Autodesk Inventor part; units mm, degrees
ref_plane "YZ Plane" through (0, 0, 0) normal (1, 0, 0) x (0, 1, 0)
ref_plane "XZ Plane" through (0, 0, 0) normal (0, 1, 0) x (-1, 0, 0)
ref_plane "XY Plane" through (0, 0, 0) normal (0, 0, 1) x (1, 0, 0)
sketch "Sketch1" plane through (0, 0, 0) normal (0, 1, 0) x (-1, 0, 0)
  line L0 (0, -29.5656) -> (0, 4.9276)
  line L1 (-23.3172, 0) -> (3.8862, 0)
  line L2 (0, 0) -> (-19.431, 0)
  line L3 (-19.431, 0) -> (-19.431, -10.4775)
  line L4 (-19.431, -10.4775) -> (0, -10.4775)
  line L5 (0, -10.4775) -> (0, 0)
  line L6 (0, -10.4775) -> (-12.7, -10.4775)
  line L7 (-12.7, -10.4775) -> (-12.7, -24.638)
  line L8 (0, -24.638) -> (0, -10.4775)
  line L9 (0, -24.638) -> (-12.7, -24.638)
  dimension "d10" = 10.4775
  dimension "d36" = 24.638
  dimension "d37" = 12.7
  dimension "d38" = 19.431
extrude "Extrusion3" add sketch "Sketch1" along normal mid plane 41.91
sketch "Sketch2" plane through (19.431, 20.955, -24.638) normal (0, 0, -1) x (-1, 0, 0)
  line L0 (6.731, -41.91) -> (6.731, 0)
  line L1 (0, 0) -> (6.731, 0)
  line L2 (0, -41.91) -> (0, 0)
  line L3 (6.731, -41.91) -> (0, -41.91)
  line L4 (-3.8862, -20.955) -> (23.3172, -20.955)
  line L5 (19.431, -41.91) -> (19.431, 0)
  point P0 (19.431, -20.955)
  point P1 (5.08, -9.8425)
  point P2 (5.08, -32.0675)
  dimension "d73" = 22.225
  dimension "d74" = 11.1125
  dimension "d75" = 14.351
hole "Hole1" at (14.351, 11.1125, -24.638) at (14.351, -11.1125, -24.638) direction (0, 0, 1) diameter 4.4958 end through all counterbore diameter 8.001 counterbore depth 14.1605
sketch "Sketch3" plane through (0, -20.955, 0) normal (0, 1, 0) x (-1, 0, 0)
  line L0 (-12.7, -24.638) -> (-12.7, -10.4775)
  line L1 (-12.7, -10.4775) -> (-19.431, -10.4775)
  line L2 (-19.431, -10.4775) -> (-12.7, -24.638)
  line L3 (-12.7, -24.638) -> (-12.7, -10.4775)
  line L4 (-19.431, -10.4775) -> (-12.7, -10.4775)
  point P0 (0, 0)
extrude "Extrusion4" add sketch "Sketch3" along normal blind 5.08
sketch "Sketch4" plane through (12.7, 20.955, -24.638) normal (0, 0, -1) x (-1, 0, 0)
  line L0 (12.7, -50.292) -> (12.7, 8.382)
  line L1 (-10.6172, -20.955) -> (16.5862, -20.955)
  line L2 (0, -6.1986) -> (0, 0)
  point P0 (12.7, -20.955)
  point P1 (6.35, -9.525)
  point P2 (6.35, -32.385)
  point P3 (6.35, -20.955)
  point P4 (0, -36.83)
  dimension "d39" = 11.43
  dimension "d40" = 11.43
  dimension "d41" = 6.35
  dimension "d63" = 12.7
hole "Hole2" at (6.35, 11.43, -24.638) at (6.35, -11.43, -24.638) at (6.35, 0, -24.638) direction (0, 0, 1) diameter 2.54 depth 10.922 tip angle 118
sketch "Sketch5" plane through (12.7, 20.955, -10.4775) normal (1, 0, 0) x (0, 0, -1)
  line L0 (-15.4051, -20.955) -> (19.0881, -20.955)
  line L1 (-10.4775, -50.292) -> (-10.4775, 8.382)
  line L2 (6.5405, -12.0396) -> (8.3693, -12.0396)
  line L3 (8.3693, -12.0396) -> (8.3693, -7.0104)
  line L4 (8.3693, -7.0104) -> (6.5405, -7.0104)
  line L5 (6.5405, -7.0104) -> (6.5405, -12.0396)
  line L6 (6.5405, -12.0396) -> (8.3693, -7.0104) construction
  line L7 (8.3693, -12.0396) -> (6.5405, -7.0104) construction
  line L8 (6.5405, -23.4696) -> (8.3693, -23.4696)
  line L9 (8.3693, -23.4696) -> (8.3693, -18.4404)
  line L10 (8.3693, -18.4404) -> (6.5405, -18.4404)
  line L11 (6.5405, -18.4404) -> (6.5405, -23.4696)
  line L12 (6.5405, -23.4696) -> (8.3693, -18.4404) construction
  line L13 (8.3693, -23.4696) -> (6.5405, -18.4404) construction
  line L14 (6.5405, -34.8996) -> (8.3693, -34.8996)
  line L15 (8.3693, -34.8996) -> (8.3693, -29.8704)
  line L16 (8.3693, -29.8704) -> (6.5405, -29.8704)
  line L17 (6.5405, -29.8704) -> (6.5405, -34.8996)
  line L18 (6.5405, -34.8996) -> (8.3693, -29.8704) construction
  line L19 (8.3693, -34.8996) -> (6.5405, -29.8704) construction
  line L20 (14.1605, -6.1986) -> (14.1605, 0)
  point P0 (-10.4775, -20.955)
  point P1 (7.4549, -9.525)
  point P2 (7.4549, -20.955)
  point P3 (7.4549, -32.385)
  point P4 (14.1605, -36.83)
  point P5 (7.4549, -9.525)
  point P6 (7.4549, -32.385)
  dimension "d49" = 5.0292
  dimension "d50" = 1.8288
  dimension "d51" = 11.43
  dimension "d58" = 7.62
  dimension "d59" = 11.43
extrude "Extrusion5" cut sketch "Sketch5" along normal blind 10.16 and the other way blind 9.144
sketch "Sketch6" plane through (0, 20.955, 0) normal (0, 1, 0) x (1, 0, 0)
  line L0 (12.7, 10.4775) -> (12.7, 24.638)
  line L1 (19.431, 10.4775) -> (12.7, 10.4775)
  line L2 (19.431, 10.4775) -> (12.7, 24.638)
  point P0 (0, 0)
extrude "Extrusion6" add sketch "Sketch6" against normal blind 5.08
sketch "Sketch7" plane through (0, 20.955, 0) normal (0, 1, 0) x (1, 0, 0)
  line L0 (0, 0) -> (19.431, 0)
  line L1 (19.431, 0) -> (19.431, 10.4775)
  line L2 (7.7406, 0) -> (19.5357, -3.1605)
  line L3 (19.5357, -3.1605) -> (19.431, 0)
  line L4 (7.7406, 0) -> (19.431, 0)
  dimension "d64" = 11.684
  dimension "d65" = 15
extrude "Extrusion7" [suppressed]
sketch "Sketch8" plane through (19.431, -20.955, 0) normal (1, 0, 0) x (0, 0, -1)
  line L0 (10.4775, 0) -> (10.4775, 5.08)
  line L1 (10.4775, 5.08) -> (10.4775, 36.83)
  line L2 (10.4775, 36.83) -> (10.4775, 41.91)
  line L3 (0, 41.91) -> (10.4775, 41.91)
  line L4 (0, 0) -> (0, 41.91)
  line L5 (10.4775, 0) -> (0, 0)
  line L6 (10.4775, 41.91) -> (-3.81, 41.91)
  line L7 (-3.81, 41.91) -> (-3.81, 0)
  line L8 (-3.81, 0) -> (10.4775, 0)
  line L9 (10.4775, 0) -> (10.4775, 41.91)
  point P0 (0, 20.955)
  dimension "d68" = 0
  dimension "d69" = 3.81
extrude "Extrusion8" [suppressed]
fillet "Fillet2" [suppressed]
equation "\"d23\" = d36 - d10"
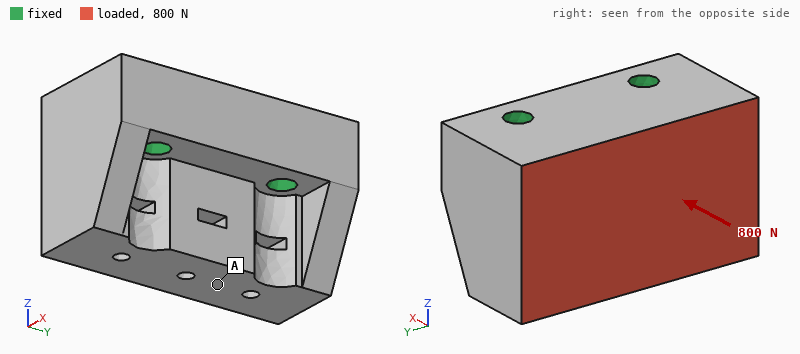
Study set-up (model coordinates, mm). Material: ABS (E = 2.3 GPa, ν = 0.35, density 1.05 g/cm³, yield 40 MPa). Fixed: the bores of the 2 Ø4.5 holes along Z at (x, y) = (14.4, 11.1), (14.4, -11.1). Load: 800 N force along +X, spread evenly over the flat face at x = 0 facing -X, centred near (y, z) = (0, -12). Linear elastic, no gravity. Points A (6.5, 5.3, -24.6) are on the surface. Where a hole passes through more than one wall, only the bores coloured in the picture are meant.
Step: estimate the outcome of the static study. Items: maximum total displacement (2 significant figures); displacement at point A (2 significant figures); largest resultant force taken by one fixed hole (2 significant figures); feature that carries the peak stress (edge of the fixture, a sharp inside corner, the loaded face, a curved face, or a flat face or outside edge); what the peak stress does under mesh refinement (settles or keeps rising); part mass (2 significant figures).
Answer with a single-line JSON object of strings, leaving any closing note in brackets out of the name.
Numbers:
{"maximum total displacement": "0.13 mm", "displacement at point A": "0.12 mm", "largest resultant force taken by one fixed hole": "400 N", "feature that carries the peak stress": "edge of the fixture", "what the peak stress does under mesh refinement": "keeps rising", "part mass": "16 g"}
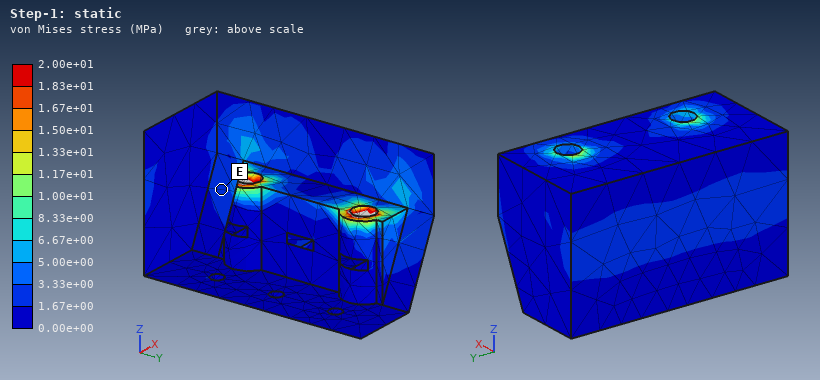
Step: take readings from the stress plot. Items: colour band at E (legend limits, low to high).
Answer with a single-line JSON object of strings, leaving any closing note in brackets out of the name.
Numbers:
{"colour band at E": "1.67e+00 to 3.33e+00 MPa"}
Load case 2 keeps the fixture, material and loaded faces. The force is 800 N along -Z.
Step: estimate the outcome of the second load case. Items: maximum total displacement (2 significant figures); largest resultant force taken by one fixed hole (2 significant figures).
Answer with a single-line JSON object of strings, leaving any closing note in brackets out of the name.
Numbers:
{"maximum total displacement": "0.23 mm", "largest resultant force taken by one fixed hole": "400 N"}
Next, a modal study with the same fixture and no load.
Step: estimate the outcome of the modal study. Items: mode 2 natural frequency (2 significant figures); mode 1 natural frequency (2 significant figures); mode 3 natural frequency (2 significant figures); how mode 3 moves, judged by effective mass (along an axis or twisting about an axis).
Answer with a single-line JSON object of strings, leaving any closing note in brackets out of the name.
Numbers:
{"mode 2 natural frequency": "5300 Hz", "mode 1 natural frequency": "3700 Hz", "mode 3 natural frequency": "6600 Hz", "how mode 3 moves, judged by effective mass": "along Y"}
